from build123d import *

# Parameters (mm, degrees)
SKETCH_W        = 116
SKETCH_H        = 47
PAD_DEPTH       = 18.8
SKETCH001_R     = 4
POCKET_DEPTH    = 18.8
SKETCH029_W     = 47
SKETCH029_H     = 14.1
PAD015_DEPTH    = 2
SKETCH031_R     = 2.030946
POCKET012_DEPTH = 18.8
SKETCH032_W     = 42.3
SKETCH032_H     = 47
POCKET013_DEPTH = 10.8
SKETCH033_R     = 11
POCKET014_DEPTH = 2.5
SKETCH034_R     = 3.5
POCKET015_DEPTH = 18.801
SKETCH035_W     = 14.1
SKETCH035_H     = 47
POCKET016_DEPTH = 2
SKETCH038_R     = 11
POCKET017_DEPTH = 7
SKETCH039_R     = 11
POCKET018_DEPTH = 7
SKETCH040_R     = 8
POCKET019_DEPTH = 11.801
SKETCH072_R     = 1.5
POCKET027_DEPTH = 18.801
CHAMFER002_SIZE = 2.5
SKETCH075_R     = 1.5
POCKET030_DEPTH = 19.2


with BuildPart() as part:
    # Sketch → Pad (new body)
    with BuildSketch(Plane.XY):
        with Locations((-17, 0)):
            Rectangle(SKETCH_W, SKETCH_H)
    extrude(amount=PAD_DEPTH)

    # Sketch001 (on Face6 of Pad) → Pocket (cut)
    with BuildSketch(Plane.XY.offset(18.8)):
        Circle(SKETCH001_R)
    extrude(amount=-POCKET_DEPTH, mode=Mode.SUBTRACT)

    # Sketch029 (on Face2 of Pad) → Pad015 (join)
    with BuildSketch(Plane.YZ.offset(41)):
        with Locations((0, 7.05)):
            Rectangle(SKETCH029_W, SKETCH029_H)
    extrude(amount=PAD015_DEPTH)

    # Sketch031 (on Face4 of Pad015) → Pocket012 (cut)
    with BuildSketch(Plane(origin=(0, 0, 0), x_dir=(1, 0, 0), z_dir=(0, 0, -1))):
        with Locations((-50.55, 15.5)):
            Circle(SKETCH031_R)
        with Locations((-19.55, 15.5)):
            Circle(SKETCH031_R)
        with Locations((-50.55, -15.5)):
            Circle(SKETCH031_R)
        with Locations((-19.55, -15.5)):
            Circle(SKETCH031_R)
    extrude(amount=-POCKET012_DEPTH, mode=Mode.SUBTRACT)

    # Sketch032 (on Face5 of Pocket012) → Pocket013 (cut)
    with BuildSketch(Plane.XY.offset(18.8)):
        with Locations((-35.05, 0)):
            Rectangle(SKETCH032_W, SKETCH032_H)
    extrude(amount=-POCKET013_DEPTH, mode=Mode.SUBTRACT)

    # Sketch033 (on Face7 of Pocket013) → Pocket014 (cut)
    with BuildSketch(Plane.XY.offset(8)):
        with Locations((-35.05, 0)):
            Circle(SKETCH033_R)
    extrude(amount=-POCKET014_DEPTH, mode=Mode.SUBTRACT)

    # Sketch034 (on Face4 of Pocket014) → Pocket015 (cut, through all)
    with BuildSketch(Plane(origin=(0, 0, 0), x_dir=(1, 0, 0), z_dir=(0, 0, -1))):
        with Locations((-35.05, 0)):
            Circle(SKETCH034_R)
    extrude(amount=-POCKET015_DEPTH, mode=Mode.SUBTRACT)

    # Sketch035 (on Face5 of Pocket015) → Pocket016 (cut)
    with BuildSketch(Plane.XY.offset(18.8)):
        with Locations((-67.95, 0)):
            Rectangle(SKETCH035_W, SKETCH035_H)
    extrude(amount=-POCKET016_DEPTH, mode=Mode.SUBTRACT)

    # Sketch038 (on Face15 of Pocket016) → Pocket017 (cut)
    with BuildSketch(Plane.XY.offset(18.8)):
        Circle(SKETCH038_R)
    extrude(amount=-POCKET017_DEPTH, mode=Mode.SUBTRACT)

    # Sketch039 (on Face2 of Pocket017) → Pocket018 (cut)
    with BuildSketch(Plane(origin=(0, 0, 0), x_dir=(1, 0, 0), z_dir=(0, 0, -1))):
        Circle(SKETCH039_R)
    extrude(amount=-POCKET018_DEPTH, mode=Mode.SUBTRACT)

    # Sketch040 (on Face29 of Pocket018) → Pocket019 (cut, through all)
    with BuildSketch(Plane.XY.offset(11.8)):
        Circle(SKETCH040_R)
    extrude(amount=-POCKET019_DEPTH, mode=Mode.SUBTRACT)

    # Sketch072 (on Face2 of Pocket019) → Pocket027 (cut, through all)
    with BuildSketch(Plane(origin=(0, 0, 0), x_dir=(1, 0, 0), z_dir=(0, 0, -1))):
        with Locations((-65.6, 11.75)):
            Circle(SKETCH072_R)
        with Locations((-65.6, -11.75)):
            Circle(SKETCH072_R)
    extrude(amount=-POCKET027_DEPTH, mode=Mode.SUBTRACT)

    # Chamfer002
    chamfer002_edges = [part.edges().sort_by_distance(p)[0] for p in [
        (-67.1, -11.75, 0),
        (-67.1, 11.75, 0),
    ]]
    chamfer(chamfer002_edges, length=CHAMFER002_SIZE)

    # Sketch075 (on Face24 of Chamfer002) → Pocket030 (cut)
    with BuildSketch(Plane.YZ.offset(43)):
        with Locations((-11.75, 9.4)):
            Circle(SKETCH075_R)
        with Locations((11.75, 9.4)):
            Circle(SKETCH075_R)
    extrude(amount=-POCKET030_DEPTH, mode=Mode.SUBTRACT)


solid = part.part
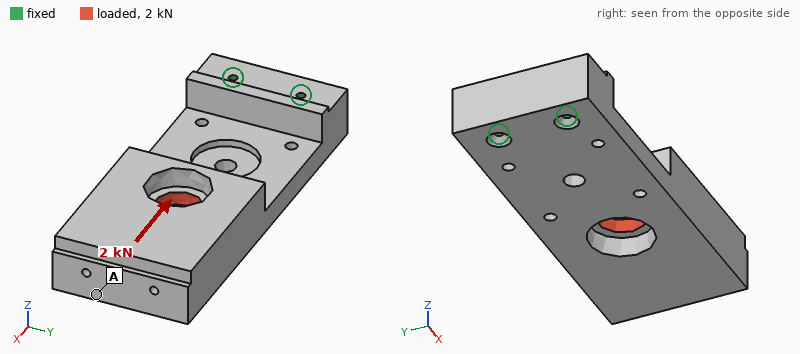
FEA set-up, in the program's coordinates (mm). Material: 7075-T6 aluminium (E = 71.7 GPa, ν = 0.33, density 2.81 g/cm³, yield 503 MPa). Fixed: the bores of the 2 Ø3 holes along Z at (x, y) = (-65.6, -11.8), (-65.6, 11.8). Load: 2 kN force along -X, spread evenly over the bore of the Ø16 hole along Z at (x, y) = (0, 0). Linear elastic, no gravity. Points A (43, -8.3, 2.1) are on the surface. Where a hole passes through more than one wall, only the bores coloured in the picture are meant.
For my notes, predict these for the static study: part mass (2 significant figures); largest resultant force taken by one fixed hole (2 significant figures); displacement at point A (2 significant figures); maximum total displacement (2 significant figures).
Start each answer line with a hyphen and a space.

- 200 g
- 1.0 kN
- 0.37 mm
- 0.37 mm
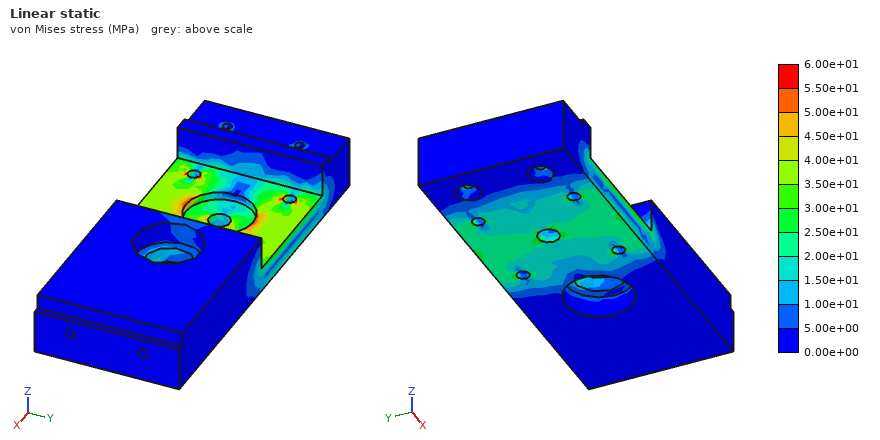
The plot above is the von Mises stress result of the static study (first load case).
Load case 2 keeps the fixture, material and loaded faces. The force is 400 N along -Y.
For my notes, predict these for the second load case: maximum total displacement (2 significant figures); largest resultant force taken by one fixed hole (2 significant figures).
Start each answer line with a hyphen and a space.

- 38 µm
- 1.1 kN
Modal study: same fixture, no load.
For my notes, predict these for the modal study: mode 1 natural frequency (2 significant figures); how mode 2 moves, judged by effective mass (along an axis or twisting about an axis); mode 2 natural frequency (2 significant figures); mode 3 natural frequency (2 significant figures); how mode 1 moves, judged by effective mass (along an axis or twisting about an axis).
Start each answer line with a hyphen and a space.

- 380 Hz
- along Y
- 1500 Hz
- 2100 Hz
- along Z
